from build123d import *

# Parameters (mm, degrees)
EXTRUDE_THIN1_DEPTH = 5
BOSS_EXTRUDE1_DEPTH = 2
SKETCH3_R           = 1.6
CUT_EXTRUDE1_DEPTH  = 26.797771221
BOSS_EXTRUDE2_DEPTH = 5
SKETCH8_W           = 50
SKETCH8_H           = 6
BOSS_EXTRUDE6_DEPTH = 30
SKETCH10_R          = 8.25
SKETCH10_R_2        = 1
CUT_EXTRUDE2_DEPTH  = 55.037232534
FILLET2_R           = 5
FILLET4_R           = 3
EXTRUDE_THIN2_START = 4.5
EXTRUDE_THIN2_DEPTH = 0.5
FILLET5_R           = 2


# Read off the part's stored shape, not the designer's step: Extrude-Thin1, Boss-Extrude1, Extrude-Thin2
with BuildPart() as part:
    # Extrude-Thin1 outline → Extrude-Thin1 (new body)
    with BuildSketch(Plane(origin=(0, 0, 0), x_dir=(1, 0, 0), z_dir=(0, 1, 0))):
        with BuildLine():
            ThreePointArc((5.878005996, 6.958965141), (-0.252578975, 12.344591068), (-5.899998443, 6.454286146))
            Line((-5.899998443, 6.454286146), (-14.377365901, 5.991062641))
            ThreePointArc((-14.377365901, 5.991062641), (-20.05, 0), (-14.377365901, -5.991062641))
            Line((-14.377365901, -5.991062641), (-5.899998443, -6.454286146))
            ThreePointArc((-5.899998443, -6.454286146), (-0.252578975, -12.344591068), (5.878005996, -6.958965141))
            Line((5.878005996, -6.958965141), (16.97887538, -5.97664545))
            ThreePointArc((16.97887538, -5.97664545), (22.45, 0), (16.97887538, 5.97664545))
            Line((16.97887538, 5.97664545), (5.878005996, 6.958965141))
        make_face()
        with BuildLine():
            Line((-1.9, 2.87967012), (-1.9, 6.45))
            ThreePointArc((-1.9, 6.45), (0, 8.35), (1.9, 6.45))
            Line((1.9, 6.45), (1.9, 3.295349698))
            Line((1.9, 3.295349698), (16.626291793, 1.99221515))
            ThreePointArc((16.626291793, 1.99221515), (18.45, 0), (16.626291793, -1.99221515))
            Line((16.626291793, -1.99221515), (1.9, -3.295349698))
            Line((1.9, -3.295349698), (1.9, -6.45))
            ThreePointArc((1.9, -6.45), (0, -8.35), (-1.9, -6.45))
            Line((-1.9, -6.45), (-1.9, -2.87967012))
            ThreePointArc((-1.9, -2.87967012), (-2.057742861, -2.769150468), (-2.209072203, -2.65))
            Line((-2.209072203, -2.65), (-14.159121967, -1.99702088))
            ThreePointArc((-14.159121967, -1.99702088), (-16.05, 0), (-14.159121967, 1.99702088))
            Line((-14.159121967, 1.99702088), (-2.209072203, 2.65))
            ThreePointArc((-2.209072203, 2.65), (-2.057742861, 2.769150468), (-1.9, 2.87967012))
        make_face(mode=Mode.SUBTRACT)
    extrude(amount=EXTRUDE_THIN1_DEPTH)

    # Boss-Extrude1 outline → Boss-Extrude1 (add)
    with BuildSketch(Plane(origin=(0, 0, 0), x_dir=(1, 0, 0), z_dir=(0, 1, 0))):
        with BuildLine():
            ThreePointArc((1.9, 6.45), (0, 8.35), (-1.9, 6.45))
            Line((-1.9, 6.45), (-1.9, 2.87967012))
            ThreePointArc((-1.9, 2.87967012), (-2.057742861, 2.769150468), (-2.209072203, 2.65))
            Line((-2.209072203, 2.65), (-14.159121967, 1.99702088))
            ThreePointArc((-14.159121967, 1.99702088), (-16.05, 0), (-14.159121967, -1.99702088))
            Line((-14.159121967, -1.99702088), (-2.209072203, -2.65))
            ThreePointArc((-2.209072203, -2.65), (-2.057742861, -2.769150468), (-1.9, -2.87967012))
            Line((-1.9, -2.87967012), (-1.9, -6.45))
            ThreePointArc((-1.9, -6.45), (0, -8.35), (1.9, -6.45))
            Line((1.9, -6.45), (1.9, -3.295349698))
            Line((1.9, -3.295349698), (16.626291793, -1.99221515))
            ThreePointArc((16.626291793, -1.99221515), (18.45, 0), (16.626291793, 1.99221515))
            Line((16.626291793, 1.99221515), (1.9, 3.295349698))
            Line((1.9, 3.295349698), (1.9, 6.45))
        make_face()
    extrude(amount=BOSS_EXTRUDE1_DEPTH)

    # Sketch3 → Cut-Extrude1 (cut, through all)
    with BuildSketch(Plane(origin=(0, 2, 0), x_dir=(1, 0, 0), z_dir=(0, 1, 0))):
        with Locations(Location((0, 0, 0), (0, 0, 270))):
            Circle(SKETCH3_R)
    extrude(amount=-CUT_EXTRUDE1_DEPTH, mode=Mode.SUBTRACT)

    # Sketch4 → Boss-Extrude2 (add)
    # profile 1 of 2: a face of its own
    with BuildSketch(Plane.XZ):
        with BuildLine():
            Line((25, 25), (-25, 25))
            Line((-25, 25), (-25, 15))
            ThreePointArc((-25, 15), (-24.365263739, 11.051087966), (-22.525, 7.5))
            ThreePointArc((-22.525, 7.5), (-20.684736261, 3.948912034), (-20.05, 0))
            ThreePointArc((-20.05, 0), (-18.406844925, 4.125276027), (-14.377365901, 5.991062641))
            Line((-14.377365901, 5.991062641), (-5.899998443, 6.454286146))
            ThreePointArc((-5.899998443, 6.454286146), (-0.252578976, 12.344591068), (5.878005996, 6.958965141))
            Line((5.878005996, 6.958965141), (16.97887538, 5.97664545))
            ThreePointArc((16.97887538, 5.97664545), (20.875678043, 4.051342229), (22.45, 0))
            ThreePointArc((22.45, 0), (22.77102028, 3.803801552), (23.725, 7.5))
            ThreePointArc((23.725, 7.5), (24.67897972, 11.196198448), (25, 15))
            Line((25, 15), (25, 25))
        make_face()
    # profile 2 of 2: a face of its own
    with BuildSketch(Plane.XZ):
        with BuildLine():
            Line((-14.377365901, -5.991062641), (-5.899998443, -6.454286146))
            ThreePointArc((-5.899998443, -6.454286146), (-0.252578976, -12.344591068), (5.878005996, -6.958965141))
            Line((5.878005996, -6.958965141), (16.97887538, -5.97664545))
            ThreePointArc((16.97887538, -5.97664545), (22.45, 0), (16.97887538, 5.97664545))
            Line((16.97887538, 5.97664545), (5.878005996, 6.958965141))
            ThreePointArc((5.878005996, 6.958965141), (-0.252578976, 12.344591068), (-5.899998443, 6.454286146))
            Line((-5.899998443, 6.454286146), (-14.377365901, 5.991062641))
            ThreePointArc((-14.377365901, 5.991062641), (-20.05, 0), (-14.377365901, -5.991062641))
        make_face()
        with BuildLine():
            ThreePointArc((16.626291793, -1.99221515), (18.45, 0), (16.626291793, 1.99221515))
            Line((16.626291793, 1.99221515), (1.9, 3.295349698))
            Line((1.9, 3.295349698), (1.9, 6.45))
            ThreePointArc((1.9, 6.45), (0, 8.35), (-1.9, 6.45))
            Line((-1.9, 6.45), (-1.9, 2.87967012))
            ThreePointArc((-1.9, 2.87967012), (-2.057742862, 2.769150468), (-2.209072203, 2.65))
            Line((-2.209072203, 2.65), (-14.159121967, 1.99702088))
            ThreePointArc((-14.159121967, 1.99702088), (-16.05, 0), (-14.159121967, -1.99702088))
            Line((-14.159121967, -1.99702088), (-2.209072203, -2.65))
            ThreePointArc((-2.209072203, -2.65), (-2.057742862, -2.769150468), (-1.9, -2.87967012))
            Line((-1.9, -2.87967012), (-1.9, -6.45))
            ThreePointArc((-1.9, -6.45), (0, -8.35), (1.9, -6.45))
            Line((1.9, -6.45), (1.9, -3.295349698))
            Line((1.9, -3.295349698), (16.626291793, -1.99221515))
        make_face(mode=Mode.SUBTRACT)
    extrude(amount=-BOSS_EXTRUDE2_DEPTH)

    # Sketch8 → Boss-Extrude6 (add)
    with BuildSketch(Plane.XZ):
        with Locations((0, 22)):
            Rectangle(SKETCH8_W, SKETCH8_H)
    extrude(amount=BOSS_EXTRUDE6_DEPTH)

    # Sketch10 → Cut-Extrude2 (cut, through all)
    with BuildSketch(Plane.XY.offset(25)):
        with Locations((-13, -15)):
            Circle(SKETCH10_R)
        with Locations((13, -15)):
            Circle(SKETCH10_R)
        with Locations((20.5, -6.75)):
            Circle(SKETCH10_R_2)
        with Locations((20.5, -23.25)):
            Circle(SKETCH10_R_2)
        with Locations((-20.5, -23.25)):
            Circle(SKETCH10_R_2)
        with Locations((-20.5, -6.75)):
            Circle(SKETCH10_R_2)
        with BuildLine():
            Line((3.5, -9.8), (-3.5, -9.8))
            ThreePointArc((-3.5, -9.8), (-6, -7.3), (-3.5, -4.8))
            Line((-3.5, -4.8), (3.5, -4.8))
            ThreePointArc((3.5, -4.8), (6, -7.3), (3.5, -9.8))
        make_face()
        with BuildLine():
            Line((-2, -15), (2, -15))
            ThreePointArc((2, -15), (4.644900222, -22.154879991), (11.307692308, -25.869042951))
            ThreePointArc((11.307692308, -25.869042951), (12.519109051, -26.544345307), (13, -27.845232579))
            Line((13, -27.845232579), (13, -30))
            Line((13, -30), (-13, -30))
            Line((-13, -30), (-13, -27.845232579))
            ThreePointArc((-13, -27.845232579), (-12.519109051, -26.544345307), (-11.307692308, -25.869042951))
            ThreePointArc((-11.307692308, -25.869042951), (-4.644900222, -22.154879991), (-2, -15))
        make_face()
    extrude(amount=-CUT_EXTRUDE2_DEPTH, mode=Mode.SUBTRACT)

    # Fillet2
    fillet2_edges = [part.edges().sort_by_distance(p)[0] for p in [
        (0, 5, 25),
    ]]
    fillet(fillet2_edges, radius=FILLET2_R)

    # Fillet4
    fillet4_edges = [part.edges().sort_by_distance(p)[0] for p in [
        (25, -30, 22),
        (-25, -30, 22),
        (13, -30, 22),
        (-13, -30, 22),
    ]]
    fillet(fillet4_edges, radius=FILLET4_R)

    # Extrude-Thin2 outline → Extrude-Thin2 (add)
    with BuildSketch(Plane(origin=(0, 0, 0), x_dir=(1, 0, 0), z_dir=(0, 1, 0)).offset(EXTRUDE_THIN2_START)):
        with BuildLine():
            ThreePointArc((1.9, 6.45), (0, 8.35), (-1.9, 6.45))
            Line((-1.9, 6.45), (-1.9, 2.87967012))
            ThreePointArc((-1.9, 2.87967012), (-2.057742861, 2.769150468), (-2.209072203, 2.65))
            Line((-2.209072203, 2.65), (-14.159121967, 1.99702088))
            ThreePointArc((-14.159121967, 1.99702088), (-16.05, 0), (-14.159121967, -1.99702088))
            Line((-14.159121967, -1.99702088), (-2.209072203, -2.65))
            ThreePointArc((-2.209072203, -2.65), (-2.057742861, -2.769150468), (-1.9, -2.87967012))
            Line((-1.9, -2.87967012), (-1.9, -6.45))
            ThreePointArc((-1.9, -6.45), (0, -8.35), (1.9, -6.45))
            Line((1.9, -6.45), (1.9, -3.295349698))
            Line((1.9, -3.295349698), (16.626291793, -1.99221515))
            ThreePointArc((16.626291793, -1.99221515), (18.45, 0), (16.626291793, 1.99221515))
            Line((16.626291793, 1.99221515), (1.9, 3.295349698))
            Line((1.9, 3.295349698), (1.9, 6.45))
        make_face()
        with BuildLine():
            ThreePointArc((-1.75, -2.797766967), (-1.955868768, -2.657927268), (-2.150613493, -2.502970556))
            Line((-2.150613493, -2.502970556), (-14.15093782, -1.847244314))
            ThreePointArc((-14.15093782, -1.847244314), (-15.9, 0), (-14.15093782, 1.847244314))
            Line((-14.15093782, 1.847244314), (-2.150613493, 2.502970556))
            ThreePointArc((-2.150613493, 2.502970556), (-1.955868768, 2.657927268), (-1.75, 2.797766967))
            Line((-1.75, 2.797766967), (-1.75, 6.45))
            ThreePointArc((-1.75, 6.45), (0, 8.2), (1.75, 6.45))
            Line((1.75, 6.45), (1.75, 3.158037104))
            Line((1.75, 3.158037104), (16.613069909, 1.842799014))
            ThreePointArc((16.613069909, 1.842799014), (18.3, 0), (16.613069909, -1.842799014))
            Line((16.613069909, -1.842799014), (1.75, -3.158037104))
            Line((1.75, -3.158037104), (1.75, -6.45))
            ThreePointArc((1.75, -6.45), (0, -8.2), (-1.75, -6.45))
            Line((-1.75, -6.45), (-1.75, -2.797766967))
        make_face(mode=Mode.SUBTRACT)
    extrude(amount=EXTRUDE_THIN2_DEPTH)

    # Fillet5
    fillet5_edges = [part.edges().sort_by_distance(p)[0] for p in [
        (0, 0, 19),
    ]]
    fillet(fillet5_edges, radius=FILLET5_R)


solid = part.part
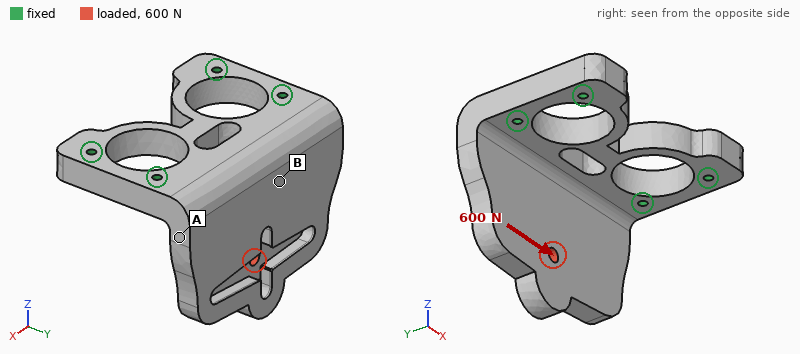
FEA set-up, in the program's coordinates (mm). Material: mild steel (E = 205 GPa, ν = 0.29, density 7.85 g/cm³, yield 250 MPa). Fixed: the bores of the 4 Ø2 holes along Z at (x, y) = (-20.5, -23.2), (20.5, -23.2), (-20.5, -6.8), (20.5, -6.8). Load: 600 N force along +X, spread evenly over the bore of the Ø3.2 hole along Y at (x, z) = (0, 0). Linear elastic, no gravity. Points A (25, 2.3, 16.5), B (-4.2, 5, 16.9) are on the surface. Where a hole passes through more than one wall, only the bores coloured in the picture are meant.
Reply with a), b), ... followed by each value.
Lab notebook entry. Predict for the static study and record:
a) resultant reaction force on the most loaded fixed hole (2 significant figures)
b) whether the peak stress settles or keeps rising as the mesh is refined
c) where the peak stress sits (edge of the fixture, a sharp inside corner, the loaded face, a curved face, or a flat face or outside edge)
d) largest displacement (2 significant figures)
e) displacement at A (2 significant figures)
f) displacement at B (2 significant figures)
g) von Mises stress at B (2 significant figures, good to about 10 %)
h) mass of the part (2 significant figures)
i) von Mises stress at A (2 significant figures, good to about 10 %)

a) 450 N
b) keeps rising
c) edge of the fixture
d) 6.7 µm
e) 3.3 µm
f) 1.1 µm
g) 4.1 MPa
h) 90 g
i) 9.0 MPa
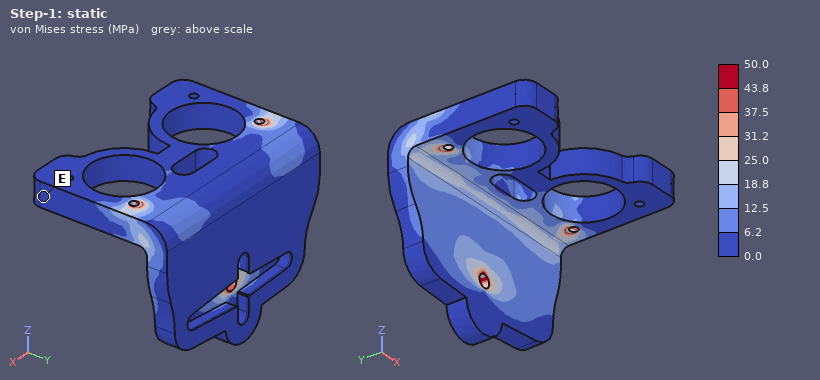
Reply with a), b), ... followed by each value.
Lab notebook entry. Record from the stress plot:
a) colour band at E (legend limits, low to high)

a) 0.0 to 6.2 MPa
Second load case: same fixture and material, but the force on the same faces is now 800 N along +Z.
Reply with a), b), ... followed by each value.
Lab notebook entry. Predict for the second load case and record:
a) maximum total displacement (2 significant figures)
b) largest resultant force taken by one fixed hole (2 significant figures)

a) 9.8 µm
b) 430 N
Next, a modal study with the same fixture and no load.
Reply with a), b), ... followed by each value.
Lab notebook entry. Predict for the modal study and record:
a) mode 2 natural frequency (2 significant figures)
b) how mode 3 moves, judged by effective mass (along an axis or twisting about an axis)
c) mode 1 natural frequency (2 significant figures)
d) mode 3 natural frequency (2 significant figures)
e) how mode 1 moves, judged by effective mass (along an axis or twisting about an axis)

a) 8100 Hz
b) along Z
c) 3500 Hz
d) 10 kHz
e) along Y
